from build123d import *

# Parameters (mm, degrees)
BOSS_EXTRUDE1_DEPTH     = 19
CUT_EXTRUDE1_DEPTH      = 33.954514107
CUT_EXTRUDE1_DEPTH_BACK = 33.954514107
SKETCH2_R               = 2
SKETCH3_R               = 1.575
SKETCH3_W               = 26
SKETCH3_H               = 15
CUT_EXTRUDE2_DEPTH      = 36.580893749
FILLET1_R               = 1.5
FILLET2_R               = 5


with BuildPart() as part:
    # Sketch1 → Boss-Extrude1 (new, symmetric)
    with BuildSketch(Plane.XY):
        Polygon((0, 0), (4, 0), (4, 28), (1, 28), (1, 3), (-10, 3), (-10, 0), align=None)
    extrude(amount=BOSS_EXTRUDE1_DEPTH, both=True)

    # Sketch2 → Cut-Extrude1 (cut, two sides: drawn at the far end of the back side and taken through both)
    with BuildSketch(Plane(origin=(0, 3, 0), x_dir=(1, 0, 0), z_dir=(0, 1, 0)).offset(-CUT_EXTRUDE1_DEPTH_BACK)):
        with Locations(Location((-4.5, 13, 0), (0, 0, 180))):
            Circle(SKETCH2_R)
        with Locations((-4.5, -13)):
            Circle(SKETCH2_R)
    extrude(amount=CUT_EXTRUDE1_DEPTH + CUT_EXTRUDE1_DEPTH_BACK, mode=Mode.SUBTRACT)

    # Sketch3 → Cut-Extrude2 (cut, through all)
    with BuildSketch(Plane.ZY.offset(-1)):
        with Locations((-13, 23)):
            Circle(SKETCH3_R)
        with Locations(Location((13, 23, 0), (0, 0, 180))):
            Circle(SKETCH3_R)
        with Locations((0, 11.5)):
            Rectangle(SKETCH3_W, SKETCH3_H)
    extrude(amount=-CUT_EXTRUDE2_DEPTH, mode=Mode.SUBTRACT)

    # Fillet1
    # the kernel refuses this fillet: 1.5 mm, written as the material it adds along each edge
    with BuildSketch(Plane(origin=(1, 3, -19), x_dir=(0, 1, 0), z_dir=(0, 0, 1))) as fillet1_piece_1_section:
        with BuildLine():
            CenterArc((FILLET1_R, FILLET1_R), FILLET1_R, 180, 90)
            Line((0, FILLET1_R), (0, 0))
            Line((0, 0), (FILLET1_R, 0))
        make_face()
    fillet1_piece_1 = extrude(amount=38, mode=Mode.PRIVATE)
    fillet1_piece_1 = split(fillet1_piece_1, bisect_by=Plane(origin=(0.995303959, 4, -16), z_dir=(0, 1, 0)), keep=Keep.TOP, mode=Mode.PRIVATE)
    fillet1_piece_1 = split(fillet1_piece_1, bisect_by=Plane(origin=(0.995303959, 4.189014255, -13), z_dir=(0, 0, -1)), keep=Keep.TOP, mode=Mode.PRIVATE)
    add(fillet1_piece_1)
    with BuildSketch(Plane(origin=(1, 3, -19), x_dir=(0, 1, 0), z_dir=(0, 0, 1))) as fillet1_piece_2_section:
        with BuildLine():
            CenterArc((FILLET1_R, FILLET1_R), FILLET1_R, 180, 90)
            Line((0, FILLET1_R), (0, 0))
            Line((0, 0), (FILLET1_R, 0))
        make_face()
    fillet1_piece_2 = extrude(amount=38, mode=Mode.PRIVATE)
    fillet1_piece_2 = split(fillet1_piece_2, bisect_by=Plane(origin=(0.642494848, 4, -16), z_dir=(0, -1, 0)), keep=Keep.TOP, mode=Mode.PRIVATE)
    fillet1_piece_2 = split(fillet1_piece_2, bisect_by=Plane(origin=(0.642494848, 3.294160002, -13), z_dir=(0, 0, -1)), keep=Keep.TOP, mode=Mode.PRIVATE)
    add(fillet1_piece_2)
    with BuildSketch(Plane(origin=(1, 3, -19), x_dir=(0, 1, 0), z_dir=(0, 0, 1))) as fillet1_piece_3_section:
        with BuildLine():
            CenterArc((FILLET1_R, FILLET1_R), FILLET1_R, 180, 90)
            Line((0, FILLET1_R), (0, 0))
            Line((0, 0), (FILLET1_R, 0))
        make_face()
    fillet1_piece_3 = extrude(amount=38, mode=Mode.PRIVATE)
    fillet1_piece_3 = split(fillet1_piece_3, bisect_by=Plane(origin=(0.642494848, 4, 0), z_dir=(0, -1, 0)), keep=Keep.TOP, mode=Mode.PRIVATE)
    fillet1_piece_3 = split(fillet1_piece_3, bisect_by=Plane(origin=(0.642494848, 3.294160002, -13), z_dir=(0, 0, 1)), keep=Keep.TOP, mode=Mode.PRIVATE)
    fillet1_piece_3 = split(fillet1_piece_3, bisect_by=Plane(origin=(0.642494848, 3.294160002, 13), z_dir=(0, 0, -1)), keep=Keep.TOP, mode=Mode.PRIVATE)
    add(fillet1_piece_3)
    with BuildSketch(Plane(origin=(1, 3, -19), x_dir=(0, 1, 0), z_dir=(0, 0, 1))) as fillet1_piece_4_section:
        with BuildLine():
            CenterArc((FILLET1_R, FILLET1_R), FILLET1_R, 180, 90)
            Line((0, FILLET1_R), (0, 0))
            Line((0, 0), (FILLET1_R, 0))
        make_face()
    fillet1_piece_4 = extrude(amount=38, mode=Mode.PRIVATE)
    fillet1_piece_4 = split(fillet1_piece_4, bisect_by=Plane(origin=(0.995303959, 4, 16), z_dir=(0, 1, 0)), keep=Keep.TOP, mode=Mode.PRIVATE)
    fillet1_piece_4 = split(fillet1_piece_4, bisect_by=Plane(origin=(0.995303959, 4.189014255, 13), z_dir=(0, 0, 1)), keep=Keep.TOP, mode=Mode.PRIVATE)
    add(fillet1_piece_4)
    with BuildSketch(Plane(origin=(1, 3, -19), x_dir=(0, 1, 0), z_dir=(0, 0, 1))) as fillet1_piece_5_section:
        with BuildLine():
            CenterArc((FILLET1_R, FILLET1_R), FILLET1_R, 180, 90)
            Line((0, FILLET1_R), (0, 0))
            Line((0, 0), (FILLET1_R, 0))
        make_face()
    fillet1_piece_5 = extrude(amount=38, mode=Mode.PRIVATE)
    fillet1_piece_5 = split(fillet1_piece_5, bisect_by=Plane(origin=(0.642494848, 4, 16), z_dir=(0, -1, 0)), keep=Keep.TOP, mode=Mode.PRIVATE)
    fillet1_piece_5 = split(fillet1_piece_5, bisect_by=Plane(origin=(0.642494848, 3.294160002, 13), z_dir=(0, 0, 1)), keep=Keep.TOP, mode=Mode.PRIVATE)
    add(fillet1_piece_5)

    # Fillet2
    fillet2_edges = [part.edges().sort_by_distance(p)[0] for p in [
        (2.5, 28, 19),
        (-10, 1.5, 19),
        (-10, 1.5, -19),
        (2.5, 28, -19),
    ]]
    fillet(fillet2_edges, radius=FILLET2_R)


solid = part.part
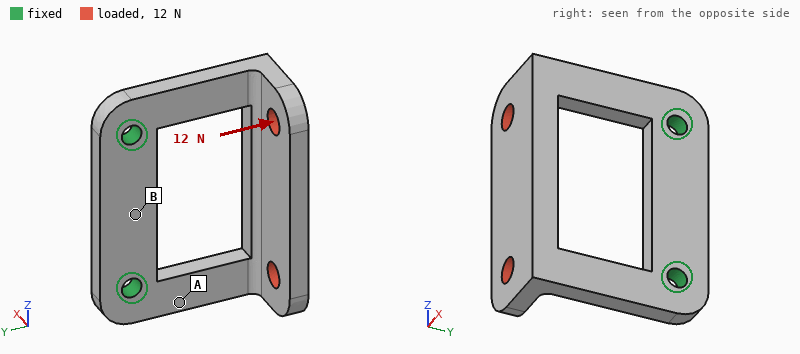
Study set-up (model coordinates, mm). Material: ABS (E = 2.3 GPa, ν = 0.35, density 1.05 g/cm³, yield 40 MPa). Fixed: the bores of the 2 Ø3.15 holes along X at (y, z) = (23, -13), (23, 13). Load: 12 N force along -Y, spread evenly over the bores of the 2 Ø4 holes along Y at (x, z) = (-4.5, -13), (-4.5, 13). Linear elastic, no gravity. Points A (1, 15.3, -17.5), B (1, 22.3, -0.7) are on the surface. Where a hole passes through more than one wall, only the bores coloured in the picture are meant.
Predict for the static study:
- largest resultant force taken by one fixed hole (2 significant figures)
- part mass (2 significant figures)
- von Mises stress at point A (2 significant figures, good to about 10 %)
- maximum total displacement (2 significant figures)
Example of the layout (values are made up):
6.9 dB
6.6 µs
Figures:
6.1 N
3.3 g
4.8 MPa
0.49 mm
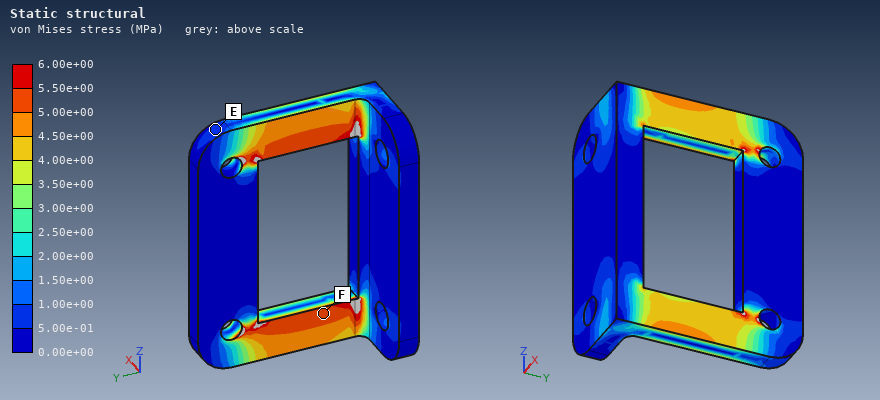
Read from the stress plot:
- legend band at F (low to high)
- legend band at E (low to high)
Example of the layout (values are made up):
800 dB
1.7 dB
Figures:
5.00e+00 to 5.50e+00 MPa
5.00e-01 to 1.00e+00 MPa
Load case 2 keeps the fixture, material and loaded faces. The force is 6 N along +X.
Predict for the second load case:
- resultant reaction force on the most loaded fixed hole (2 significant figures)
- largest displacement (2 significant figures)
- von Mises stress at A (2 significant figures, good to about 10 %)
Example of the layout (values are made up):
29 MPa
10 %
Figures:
3.0 N
0.41 mm
4.5 MPa
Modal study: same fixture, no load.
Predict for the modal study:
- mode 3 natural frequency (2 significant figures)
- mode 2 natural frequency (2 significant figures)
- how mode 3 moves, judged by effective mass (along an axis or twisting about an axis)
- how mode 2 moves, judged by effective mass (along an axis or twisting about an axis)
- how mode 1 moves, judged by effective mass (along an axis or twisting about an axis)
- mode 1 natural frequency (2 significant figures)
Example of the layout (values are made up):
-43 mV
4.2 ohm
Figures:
1600 Hz
1100 Hz
along Z
along Z
along X
490 Hz
